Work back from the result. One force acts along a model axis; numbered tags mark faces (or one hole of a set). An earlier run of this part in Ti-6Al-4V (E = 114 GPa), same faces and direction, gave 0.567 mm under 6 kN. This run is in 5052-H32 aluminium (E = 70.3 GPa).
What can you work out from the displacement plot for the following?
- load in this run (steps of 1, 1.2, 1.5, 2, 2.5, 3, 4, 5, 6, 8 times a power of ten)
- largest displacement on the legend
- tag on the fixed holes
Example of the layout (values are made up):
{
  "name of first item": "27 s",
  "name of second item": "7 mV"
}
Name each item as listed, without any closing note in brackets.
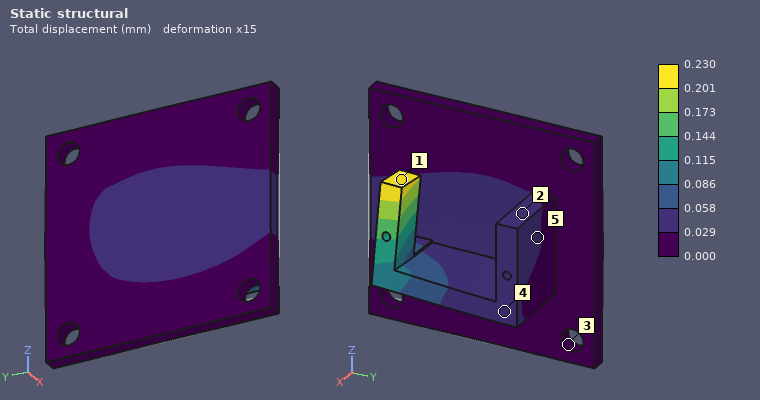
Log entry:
{
  "load in this run": "1.5 kN",
  "largest displacement on the legend": "0.230 mm",
  "tag on the fixed holes": "3"
}
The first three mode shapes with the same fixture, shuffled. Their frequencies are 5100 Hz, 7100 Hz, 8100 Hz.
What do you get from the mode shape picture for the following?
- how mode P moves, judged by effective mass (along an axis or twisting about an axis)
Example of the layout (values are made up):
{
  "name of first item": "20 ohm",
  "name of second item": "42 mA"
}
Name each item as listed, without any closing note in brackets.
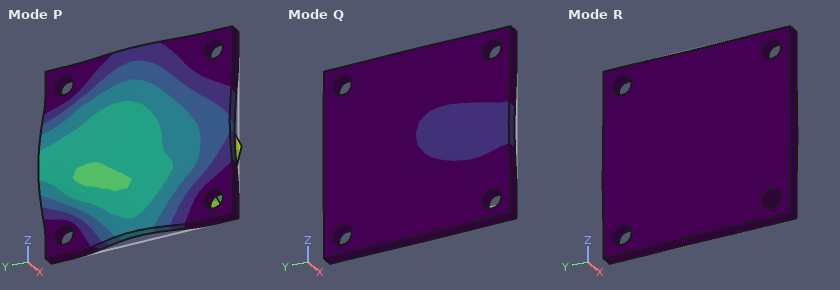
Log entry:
{
  "how mode P moves, judged by effective mass": "along X"
}
